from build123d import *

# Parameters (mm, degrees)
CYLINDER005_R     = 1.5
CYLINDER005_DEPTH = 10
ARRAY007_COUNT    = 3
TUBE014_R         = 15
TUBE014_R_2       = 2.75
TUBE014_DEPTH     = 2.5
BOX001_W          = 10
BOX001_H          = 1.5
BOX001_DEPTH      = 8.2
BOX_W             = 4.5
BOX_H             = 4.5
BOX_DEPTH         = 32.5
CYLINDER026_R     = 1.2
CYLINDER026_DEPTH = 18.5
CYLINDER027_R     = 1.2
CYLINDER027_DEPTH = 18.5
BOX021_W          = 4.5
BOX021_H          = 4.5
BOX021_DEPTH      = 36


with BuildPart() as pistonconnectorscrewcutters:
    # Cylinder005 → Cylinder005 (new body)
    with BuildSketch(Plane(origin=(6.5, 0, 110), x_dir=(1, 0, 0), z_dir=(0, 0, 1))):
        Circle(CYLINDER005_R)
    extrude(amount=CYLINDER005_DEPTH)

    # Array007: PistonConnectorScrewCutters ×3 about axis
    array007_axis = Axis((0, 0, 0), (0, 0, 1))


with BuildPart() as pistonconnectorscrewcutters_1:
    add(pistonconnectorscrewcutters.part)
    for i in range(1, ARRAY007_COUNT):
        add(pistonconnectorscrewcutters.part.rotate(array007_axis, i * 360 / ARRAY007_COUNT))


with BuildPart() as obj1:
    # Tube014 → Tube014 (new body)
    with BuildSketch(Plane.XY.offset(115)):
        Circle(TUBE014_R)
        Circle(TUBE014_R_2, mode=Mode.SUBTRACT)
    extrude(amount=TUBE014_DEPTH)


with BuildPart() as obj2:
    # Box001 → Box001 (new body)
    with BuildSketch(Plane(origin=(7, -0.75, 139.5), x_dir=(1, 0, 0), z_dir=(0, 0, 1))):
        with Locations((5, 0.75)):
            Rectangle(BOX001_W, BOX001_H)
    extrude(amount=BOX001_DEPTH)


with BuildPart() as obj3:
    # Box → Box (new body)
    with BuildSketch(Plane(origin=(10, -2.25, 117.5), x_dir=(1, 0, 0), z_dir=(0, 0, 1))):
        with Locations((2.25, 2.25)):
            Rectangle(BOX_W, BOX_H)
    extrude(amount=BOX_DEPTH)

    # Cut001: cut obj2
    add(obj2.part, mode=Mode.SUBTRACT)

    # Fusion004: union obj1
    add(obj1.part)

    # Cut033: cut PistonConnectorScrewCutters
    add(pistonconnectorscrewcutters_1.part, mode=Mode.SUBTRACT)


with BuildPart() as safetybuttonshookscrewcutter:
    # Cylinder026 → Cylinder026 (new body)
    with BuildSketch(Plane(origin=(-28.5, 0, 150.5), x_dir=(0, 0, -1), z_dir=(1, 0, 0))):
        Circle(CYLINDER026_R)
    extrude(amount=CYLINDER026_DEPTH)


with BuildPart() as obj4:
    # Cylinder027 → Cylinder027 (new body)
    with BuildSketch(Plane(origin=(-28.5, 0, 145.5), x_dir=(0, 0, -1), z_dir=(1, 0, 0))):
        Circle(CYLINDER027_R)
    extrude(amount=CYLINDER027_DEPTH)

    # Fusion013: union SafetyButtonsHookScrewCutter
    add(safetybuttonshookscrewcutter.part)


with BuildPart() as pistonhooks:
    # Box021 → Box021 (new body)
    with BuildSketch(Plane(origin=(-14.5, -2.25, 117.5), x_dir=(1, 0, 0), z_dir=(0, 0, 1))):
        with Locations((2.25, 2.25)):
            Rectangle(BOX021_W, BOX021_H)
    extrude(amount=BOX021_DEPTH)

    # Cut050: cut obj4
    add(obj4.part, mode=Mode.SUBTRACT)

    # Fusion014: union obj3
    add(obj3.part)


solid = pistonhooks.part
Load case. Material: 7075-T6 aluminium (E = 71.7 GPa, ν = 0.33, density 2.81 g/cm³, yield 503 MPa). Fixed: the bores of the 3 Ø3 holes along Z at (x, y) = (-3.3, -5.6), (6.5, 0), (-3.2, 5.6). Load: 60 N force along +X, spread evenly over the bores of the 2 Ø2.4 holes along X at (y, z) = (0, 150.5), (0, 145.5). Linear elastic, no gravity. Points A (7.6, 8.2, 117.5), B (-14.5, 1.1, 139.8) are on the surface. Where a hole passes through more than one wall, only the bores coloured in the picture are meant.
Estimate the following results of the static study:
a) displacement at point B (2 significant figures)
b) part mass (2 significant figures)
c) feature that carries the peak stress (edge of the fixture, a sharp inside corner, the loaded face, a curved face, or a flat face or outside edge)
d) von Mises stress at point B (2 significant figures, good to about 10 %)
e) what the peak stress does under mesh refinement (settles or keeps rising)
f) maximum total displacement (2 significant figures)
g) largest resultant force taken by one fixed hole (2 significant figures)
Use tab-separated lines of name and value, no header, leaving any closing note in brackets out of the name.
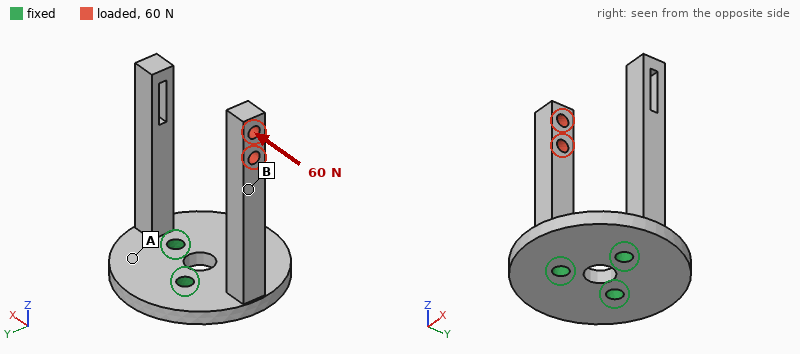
displacement at point B	0.36 mm
part mass	8.3 g
feature that carries the peak stress	edge of the fixture
von Mises stress at point B	33 MPa
what the peak stress does under mesh refinement	keeps rising
maximum total displacement	0.64 mm
largest resultant force taken by one fixed hole	38 N
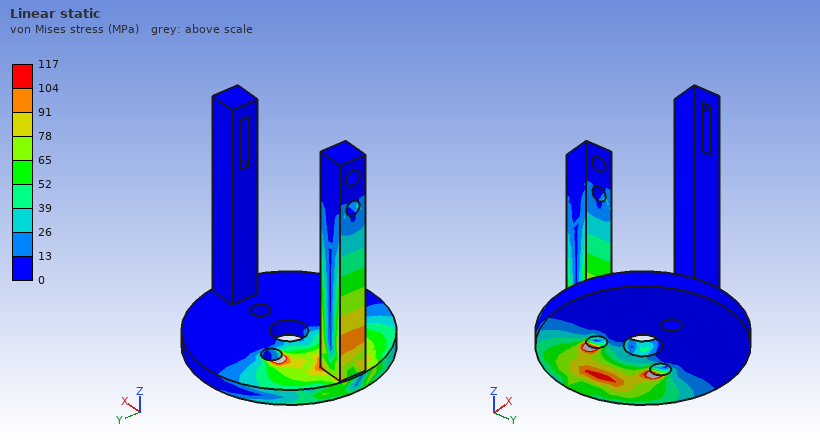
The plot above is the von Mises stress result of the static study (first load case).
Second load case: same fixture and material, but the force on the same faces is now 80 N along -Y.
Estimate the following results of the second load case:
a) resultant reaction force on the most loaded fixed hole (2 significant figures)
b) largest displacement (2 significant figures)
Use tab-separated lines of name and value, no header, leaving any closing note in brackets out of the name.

resultant reaction force on the most loaded fixed hole	230 N
largest displacement	0.61 mm
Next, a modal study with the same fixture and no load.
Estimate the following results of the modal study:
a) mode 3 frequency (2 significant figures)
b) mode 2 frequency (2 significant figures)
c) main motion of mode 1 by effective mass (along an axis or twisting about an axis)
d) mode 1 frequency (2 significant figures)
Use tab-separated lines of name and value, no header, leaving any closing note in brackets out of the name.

mode 3 frequency	2500 Hz
mode 2 frequency	2300 Hz
main motion of mode 1 by effective mass	along X
mode 1 frequency	1900 Hz
